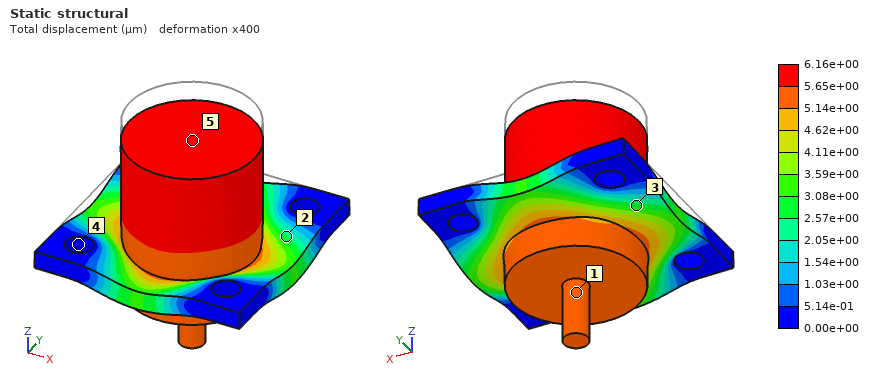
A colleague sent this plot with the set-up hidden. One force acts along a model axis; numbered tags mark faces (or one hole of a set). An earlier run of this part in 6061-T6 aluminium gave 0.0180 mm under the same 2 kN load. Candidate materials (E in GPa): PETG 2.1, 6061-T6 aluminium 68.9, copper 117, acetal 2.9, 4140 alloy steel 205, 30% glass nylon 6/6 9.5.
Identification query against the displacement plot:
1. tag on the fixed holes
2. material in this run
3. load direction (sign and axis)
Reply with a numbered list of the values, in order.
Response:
1. 4
2. 4140 alloy steel
3. -Z
